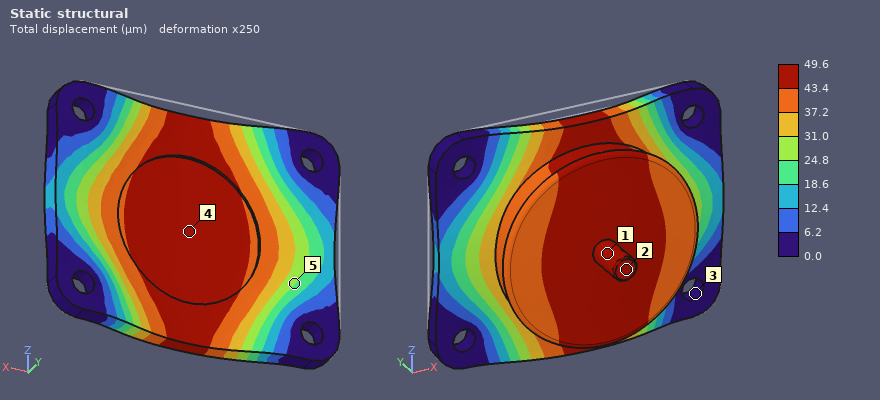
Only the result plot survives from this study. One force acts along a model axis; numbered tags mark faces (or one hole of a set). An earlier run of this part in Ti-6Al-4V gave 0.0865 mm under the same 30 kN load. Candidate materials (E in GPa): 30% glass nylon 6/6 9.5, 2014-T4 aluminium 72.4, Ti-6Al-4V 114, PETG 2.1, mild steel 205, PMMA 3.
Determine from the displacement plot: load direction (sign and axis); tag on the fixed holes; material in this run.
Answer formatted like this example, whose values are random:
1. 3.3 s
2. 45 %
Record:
1. -Y
2. 3
3. mild steel
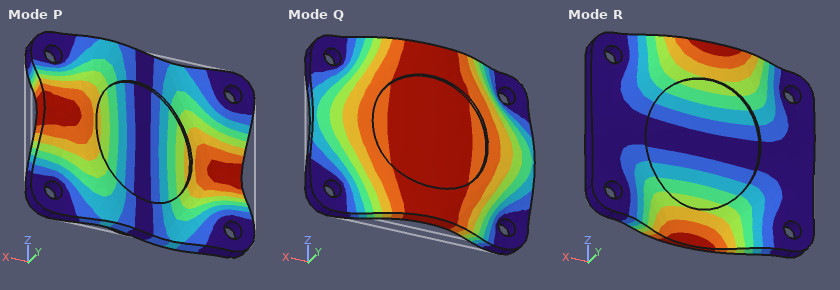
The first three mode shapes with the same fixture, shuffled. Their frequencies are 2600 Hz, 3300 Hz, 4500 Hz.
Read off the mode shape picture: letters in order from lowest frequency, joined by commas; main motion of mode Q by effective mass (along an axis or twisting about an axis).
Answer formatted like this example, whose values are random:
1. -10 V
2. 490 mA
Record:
1. Q, R, P
2. along Y
